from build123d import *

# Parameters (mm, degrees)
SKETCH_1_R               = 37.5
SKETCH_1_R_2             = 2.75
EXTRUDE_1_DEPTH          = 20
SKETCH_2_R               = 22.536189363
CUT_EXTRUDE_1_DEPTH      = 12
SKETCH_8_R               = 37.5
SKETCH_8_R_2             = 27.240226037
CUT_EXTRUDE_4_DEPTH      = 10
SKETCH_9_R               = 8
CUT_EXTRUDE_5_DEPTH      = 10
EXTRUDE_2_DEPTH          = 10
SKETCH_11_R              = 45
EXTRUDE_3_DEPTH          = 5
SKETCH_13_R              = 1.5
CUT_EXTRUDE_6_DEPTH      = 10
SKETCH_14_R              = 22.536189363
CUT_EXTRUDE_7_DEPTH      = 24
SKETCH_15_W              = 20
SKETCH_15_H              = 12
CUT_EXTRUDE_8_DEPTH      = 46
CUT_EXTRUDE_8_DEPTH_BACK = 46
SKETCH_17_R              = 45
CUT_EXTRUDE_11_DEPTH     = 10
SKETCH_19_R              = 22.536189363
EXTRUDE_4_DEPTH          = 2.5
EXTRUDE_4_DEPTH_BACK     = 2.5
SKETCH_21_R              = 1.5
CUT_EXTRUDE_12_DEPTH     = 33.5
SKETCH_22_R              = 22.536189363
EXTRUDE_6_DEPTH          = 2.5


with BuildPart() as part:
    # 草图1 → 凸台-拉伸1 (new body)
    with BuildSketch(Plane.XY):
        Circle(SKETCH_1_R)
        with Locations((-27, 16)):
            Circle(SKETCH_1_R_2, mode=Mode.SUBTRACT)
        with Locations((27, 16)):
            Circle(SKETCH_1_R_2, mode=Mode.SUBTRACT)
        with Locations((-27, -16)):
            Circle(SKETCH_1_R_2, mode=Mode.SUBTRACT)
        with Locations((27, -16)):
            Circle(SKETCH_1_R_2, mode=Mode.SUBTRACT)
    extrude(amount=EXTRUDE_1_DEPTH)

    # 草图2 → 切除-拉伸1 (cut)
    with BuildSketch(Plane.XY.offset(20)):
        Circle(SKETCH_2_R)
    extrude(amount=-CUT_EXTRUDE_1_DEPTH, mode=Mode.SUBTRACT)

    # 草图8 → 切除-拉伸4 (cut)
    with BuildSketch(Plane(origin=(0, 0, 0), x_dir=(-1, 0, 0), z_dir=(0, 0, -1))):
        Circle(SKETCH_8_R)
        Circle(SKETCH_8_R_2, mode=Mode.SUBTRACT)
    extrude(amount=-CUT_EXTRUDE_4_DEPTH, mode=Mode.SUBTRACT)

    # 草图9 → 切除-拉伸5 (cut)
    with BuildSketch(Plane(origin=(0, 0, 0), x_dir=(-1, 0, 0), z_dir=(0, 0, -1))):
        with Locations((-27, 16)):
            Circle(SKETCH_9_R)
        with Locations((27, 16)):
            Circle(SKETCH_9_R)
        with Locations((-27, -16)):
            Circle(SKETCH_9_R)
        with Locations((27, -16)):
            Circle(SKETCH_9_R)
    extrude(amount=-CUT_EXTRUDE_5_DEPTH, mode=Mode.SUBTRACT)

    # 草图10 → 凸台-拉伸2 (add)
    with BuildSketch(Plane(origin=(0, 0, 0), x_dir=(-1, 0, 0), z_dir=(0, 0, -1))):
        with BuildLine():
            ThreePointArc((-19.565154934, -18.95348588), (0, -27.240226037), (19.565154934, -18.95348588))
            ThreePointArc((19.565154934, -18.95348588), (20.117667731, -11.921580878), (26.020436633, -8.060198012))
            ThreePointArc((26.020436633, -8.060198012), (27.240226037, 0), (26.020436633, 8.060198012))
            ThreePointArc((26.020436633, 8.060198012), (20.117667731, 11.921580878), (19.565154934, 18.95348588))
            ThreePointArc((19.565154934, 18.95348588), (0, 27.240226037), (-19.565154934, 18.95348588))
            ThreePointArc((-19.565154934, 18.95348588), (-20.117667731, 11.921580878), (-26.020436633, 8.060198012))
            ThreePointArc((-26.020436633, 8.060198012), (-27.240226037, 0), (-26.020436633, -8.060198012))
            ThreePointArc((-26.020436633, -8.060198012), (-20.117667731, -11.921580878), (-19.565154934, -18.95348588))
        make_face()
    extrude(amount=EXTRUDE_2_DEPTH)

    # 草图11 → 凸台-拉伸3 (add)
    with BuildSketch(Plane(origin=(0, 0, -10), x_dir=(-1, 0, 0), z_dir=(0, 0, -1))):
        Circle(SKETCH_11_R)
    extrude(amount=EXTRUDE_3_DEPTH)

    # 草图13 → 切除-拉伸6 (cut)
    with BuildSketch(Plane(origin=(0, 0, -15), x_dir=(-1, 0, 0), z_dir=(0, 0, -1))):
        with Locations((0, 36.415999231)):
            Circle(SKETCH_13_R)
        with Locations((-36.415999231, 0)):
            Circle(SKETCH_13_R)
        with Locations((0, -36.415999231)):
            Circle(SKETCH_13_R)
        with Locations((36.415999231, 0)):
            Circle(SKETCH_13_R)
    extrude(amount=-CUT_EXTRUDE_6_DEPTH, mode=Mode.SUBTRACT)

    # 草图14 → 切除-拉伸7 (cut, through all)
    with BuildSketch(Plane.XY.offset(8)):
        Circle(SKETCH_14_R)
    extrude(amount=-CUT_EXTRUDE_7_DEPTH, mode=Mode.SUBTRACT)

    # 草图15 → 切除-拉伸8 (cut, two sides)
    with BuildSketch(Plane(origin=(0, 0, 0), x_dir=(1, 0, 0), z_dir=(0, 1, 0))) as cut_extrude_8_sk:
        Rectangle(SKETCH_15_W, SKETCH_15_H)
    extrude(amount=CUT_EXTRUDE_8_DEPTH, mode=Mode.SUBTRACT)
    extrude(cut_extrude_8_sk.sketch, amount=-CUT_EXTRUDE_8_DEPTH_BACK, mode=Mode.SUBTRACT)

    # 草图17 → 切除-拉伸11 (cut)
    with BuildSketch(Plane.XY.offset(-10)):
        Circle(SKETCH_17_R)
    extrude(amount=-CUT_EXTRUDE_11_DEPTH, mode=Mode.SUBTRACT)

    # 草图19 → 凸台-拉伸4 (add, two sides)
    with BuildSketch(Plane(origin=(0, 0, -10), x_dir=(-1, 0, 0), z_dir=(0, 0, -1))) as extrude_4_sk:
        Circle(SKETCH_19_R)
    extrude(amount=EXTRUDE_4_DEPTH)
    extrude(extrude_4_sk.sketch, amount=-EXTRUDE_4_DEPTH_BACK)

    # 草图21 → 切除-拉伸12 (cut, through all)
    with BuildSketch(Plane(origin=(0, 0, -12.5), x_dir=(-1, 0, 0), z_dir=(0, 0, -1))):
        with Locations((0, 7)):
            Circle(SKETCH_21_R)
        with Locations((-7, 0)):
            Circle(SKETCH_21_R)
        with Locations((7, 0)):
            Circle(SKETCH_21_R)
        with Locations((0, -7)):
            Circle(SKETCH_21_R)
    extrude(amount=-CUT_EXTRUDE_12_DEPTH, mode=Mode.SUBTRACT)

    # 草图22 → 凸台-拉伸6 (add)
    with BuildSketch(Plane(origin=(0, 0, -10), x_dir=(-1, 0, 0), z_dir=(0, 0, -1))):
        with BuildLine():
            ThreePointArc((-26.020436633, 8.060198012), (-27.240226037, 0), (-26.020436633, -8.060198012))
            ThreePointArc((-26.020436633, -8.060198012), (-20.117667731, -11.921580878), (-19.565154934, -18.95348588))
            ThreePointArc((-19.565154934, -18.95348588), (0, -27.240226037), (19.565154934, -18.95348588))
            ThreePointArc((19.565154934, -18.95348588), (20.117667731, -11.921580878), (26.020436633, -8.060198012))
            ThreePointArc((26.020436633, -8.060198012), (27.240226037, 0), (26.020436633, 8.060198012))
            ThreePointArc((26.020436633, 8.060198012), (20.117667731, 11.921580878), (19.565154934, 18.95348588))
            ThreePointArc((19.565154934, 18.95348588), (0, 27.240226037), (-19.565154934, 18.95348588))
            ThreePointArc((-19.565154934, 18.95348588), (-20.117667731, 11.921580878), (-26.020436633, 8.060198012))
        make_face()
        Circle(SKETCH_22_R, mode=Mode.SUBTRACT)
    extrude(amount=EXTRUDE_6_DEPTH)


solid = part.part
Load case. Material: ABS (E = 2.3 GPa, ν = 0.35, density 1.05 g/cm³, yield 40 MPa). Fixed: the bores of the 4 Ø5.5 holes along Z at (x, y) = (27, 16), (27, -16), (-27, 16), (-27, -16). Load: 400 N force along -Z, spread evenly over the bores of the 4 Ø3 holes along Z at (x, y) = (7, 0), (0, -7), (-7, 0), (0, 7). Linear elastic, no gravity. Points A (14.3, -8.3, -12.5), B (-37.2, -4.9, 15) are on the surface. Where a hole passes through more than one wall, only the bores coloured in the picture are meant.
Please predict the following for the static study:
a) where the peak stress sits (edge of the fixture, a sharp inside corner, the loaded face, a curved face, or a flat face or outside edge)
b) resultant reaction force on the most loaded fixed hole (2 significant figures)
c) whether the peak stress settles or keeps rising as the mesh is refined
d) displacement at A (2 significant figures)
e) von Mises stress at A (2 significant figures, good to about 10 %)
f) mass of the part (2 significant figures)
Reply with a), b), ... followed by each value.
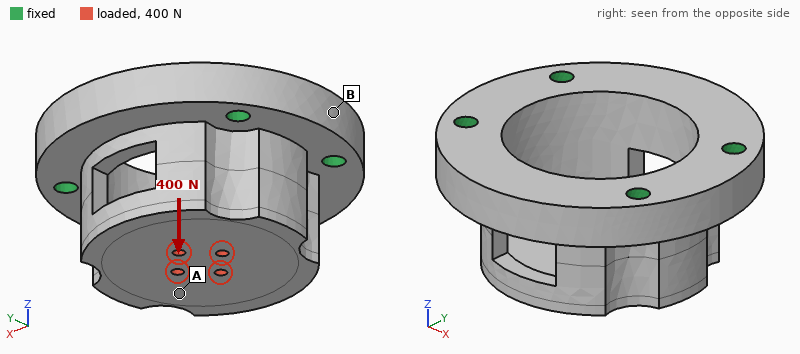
a) a sharp inside corner
b) 110 N
c) keeps rising
d) 0.10 mm
e) 4.3 MPa
f) 49 g
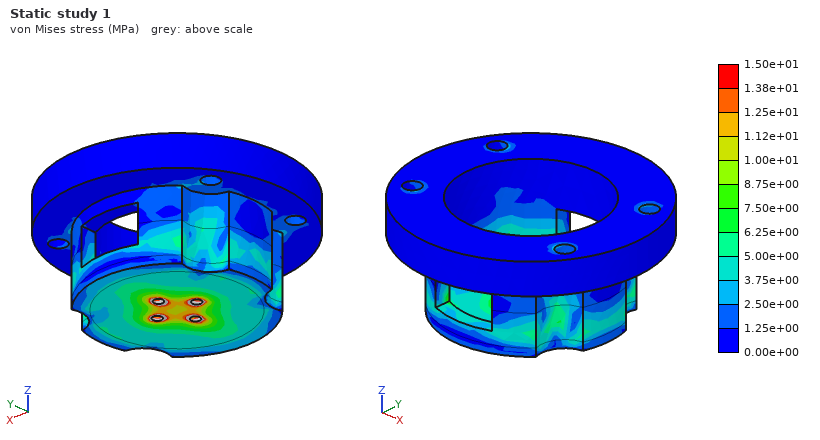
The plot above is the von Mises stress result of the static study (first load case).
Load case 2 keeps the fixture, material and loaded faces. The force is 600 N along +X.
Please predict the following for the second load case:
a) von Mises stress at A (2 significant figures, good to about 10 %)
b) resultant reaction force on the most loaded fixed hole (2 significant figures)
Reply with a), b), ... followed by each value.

a) 2.3 MPa
b) 200 N
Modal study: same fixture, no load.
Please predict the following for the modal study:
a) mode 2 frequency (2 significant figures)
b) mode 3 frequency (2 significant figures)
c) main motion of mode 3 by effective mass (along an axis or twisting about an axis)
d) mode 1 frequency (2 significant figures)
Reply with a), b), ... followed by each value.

a) 2500 Hz
b) 3400 Hz
c) along Z
d) 2500 Hz
